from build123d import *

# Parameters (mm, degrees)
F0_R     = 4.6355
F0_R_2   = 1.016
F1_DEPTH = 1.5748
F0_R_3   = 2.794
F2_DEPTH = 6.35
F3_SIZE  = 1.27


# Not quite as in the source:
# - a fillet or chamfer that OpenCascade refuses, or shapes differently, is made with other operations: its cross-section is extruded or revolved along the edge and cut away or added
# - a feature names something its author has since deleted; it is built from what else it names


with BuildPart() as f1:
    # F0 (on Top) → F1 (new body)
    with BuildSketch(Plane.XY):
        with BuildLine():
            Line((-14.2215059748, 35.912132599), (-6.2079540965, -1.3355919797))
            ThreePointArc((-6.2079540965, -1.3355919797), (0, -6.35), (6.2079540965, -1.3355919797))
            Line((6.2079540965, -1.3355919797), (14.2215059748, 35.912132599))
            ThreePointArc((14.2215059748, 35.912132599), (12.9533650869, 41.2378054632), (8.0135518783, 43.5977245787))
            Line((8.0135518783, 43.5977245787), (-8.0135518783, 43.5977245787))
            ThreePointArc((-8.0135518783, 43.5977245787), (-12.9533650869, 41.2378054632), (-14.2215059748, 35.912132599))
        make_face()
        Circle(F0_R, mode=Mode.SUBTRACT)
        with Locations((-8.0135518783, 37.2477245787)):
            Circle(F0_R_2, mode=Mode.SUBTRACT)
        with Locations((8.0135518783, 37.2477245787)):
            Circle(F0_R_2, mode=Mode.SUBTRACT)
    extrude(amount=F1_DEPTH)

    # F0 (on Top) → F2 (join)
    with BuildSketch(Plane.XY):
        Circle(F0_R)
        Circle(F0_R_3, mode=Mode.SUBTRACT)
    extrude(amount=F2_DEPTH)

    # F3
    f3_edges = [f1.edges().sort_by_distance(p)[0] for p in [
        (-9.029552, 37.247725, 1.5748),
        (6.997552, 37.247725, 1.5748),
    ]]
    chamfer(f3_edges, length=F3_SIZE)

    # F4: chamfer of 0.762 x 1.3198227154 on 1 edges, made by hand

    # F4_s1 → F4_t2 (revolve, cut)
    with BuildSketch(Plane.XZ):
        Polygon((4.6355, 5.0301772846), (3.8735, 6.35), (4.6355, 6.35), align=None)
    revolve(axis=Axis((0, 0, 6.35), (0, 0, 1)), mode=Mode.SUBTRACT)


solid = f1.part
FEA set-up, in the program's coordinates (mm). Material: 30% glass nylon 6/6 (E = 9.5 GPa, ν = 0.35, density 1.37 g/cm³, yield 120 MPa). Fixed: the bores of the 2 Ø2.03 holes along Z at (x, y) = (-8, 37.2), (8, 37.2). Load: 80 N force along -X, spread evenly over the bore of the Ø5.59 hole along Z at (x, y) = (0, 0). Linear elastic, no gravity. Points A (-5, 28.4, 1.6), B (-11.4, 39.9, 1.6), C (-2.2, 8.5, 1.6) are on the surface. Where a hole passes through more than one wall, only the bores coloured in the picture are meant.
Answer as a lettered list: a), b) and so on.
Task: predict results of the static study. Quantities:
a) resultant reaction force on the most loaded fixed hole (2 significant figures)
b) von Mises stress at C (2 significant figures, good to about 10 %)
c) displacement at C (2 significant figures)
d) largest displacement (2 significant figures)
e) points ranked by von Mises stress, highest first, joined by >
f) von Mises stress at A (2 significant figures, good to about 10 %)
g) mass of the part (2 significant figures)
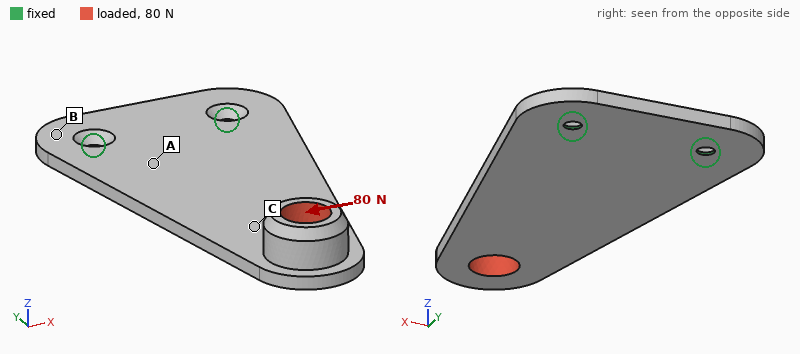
a) 180 N
b) 28 MPa
c) 0.17 mm
d) 0.51 mm
e) C > A > B
f) 16 MPa
g) 2.4 g
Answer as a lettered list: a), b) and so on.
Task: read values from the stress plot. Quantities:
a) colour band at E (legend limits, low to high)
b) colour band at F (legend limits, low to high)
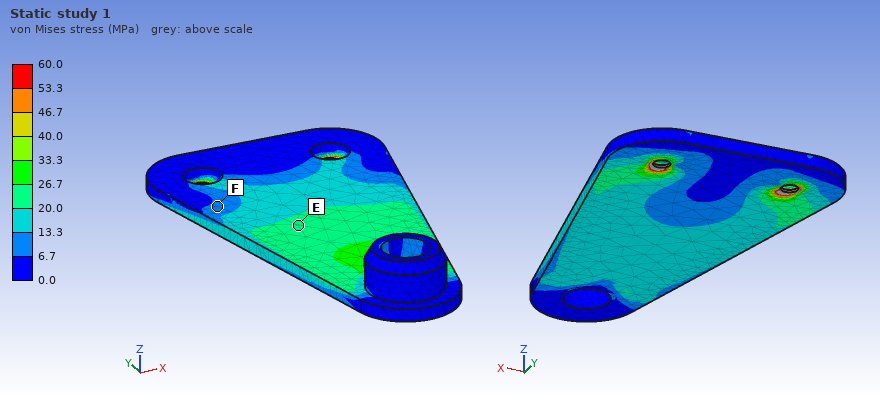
a) 20.0 to 26.7 MPa
b) 6.7 to 13.3 MPa
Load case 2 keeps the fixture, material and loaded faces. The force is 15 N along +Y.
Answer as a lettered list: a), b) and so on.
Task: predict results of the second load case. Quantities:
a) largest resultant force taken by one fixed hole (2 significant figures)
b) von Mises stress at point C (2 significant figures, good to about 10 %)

a) 7.7 N
b) 5.6 MPa
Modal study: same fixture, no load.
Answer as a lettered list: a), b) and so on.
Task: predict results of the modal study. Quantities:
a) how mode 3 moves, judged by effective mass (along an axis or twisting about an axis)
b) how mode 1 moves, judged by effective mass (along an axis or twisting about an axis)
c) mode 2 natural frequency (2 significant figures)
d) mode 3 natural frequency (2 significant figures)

a) twisting about Y
b) along Z
c) 1900 Hz
d) 2000 Hz
